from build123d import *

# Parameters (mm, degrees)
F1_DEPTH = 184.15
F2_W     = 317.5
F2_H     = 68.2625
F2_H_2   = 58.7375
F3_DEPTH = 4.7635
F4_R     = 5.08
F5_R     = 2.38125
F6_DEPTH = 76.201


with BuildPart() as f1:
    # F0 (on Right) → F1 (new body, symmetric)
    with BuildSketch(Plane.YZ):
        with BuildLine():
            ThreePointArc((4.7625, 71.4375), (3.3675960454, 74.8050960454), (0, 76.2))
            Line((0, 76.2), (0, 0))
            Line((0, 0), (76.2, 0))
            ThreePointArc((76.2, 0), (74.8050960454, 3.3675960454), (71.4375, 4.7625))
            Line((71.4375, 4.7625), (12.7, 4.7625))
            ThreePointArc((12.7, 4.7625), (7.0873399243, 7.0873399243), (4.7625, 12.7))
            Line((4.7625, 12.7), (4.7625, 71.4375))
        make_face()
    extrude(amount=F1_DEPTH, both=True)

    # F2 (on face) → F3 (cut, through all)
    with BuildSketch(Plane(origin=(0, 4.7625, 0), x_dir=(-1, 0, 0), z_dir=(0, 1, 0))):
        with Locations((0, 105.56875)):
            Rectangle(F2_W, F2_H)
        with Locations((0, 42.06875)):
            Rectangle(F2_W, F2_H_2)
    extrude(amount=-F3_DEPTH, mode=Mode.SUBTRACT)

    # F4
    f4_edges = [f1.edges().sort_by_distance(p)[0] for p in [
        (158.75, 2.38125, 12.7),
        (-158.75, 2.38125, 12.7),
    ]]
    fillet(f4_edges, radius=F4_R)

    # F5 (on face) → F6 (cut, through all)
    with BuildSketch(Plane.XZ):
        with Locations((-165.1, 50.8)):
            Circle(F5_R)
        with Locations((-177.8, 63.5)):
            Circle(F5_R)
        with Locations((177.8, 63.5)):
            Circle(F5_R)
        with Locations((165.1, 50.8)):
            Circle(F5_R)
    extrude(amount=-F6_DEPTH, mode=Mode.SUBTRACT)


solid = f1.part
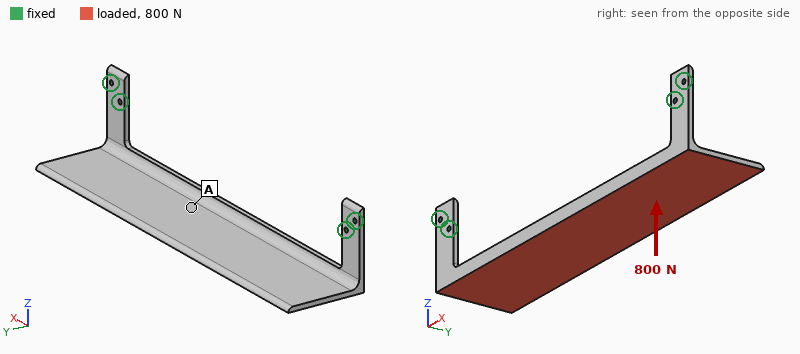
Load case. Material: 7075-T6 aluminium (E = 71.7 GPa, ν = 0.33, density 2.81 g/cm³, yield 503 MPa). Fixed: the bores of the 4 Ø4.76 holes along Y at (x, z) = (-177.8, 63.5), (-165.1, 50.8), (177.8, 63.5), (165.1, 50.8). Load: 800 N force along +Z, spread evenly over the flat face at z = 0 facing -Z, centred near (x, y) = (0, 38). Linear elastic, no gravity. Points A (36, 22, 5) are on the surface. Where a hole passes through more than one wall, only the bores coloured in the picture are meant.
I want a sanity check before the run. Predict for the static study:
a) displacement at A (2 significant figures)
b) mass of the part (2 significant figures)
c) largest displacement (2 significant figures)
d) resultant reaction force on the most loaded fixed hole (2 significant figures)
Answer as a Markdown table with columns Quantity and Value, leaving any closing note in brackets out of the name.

| Quantity | Value |
|---|---|
| displacement at A | 1.7 mm |
| mass of the part | 470 g |
| largest displacement | 4.2 mm |
| resultant reaction force on the most loaded fixed hole | 640 N |
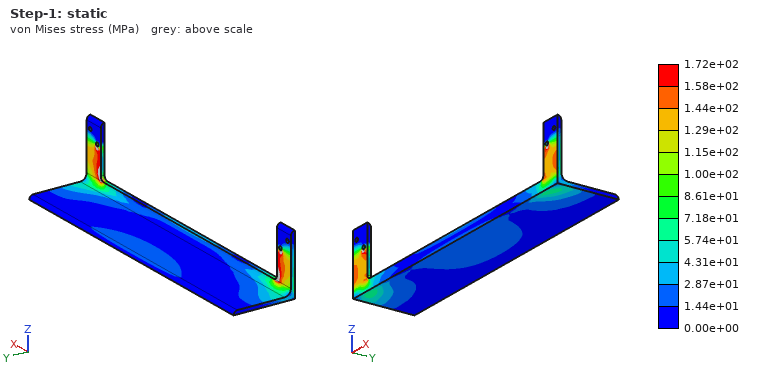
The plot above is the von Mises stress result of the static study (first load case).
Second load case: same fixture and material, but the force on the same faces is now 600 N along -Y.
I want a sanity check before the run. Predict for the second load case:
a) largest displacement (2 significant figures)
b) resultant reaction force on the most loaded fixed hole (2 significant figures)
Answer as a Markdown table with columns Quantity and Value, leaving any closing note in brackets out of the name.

| Quantity | Value |
|---|---|
| largest displacement | 2.0 mm |
| resultant reaction force on the most loaded fixed hole | 660 N |
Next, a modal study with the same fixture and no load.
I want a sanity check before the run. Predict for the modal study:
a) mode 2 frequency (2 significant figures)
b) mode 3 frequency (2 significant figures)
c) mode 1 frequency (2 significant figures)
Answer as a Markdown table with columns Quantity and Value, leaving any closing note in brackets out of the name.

| Quantity | Value |
|---|---|
| mode 2 frequency | 330 Hz |
| mode 3 frequency | 360 Hz |
| mode 1 frequency | 130 Hz |
